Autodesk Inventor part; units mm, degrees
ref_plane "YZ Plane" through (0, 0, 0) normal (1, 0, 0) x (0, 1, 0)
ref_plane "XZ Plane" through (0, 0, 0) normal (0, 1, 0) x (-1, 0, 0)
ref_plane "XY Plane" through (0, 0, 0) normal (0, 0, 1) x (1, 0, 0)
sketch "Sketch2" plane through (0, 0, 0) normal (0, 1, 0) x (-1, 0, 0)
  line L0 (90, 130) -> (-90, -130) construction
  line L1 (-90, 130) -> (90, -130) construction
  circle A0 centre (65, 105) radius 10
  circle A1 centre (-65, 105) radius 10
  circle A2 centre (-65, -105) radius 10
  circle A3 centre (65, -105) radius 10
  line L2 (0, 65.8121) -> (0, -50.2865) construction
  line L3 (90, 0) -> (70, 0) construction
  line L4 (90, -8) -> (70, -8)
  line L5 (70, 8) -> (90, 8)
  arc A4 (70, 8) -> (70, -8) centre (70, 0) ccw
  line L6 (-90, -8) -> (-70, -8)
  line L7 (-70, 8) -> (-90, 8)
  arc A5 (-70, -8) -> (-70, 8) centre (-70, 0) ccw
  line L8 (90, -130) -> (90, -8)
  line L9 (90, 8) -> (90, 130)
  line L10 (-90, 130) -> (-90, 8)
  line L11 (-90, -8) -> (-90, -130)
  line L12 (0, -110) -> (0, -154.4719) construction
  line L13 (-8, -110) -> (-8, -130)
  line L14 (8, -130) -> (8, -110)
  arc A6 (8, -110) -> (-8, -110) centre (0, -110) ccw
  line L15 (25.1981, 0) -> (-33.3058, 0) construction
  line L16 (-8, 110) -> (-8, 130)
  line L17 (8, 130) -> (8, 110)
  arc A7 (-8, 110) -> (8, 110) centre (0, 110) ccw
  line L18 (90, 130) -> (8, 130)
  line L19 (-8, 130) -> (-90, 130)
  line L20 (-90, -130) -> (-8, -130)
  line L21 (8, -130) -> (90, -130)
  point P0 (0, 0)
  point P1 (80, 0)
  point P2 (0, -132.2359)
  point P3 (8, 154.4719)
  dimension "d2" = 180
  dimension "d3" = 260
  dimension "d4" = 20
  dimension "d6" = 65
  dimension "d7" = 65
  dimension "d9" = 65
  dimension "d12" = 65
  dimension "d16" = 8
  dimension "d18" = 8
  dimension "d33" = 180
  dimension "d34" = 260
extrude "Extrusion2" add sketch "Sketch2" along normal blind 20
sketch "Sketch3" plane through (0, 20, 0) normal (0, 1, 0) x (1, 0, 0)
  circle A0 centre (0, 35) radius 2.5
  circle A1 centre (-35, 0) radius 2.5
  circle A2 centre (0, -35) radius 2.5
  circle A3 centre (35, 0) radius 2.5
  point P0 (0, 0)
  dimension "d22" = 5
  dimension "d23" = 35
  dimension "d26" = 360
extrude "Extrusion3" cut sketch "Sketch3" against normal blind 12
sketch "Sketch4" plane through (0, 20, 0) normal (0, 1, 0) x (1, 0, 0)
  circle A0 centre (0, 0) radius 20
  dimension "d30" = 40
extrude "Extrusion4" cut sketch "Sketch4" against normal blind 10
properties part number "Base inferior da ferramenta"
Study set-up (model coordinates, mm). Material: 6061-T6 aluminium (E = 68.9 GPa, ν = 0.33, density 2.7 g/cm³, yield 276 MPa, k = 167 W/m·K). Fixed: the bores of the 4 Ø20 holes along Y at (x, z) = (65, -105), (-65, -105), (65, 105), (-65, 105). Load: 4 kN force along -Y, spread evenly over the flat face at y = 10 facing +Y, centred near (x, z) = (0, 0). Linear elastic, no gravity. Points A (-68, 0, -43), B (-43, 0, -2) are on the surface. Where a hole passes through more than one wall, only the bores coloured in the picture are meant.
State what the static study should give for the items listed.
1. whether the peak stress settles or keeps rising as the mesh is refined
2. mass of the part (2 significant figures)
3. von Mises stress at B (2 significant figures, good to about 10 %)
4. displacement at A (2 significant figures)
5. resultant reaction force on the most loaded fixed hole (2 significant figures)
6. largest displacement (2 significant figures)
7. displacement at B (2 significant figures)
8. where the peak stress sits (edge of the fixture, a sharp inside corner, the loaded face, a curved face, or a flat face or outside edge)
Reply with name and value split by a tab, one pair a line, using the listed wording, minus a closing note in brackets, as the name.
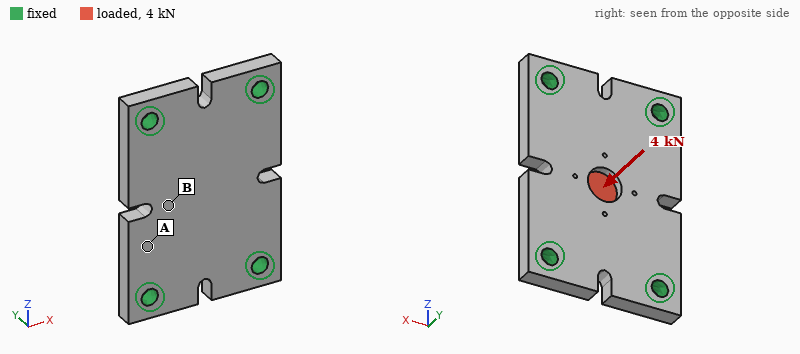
whether the peak stress settles or keeps rising as the mesh is refined	keeps rising
mass of the part	2.3 kg
von Mises stress at B	9.2 MPa
displacement at A	16 µm
resultant reaction force on the most loaded fixed hole	1.1 kN
largest displacement	47 µm
displacement at B	33 µm
where the peak stress sits	a sharp inside corner
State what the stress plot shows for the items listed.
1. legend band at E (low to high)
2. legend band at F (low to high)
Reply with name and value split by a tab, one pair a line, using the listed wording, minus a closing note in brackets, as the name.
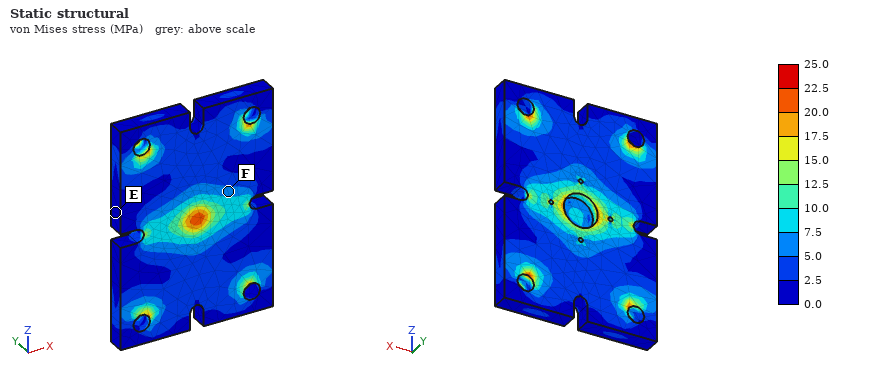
legend band at E	0.0 to 2.5 MPa
legend band at F	5.0 to 7.5 MPa
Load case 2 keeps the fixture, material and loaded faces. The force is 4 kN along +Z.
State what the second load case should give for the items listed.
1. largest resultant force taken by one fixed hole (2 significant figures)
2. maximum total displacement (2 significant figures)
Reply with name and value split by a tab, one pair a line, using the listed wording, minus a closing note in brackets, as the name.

largest resultant force taken by one fixed hole	1.1 kN
maximum total displacement	3.6 µm
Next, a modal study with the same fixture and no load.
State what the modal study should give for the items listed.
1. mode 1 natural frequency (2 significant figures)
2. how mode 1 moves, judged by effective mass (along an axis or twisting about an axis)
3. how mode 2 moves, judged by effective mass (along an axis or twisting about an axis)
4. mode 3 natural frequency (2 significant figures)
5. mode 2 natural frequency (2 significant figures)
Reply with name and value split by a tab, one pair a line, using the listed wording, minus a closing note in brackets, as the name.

mode 1 natural frequency	2100 Hz
how mode 1 moves, judged by effective mass	along Y
how mode 2 moves, judged by effective mass	twisting about Z
mode 3 natural frequency	4700 Hz
mode 2 natural frequency	2900 Hz
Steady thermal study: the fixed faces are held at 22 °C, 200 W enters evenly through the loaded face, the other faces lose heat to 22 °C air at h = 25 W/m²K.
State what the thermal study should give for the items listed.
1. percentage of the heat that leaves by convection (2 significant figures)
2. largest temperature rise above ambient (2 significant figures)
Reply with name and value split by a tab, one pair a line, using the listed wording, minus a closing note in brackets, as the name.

percentage of the heat that leaves by convection	10 %
largest temperature rise above ambient	36 K
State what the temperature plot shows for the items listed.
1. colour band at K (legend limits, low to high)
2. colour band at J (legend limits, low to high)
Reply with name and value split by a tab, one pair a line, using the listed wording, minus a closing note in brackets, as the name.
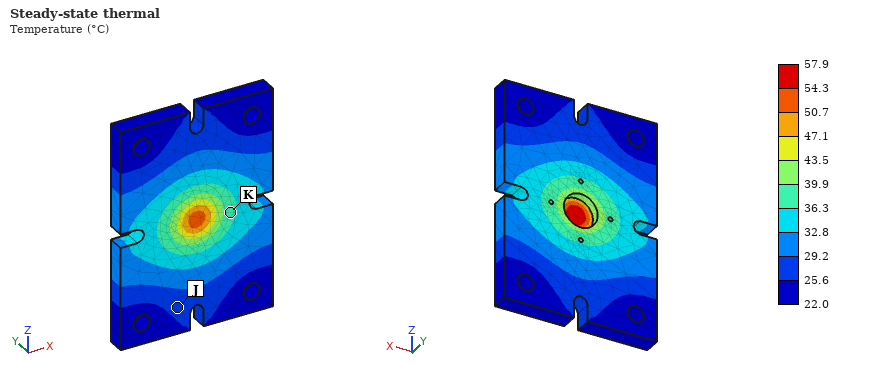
colour band at K	36.3 to 39.9 °C
colour band at J	25.6 to 29.2 °C
